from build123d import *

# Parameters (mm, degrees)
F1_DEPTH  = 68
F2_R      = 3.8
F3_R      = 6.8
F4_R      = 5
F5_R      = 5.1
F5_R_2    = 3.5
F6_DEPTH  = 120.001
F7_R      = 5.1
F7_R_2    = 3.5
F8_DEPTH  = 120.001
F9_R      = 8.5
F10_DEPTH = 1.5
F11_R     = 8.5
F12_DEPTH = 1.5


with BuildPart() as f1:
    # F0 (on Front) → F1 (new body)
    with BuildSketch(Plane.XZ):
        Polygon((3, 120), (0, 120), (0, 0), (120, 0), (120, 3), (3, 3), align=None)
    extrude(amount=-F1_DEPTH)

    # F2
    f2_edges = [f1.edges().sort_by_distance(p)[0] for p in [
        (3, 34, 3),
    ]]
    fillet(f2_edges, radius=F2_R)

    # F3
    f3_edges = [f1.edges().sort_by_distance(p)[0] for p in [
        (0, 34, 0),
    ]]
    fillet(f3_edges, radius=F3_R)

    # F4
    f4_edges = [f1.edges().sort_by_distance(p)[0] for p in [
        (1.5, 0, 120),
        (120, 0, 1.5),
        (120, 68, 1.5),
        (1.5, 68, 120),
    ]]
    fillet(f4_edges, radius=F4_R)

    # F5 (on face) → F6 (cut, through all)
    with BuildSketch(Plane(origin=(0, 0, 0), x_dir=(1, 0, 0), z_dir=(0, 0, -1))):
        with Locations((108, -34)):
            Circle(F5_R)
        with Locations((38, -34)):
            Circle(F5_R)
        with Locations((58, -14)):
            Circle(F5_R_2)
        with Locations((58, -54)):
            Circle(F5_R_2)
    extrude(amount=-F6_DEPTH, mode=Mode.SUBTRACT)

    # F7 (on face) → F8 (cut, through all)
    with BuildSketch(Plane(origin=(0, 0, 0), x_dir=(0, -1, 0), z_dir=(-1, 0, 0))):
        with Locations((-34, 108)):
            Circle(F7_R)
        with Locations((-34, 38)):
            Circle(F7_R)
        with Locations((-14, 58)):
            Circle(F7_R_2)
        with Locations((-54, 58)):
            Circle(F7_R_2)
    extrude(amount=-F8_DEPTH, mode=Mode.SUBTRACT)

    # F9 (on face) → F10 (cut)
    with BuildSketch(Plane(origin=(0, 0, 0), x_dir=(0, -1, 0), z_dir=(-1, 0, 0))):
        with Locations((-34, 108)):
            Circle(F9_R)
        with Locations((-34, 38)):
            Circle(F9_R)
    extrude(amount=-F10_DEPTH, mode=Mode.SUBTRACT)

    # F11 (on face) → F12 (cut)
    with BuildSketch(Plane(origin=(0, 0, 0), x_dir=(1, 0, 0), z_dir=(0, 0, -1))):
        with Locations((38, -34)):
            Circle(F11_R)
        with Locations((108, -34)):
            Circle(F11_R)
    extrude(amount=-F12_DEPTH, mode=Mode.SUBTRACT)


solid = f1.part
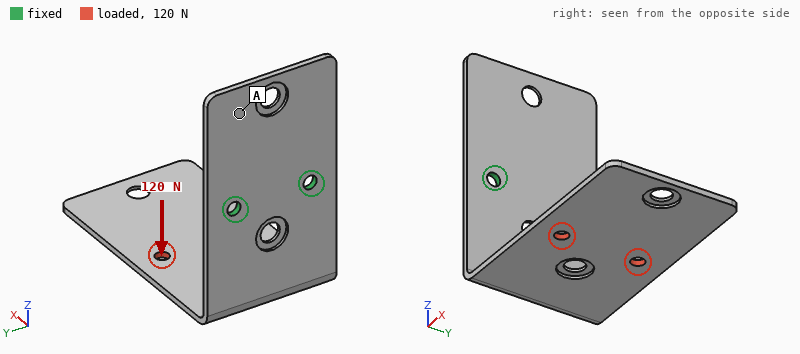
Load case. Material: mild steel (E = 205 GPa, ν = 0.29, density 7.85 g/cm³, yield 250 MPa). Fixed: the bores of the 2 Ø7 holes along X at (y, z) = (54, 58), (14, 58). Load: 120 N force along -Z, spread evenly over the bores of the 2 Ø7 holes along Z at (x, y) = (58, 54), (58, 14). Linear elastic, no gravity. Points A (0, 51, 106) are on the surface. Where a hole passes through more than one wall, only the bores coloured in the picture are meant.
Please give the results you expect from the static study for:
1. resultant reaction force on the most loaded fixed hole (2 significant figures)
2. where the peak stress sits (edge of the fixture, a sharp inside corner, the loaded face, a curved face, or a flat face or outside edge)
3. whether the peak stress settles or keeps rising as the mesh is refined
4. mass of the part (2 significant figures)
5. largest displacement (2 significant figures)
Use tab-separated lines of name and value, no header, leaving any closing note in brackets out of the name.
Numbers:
resultant reaction force on the most loaded fixed hole	72 N
where the peak stress sits	edge of the fixture
whether the peak stress settles or keeps rising as the mesh is refined	keeps rising
mass of the part	360 g
largest displacement	2.1 mm
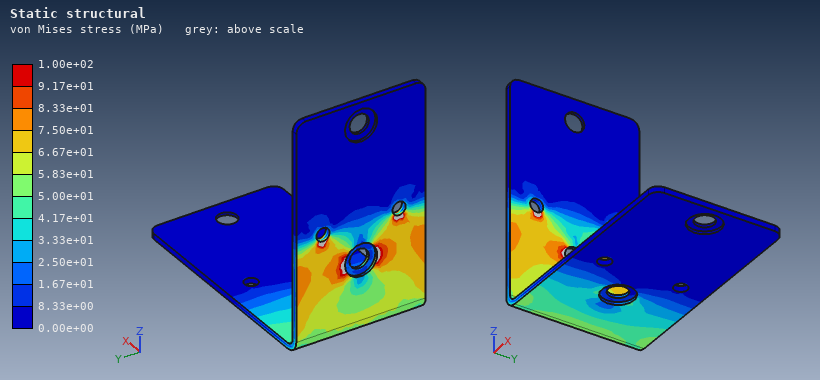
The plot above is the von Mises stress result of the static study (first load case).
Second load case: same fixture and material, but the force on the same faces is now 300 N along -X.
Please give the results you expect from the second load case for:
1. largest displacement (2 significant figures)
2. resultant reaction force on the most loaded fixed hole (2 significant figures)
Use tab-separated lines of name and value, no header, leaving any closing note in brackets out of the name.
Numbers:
largest displacement	2.0 mm
resultant reaction force on the most loaded fixed hole	160 N
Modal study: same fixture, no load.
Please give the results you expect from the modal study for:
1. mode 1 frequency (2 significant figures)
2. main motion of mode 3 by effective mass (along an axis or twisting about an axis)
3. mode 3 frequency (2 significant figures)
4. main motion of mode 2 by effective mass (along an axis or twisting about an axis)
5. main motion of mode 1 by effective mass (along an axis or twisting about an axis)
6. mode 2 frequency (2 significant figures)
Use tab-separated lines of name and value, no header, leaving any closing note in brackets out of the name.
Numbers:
mode 1 frequency	100 Hz
main motion of mode 3 by effective mass	along X
mode 3 frequency	380 Hz
main motion of mode 2 by effective mass	along Y
main motion of mode 1 by effective mass	along Z
mode 2 frequency	200 Hz
